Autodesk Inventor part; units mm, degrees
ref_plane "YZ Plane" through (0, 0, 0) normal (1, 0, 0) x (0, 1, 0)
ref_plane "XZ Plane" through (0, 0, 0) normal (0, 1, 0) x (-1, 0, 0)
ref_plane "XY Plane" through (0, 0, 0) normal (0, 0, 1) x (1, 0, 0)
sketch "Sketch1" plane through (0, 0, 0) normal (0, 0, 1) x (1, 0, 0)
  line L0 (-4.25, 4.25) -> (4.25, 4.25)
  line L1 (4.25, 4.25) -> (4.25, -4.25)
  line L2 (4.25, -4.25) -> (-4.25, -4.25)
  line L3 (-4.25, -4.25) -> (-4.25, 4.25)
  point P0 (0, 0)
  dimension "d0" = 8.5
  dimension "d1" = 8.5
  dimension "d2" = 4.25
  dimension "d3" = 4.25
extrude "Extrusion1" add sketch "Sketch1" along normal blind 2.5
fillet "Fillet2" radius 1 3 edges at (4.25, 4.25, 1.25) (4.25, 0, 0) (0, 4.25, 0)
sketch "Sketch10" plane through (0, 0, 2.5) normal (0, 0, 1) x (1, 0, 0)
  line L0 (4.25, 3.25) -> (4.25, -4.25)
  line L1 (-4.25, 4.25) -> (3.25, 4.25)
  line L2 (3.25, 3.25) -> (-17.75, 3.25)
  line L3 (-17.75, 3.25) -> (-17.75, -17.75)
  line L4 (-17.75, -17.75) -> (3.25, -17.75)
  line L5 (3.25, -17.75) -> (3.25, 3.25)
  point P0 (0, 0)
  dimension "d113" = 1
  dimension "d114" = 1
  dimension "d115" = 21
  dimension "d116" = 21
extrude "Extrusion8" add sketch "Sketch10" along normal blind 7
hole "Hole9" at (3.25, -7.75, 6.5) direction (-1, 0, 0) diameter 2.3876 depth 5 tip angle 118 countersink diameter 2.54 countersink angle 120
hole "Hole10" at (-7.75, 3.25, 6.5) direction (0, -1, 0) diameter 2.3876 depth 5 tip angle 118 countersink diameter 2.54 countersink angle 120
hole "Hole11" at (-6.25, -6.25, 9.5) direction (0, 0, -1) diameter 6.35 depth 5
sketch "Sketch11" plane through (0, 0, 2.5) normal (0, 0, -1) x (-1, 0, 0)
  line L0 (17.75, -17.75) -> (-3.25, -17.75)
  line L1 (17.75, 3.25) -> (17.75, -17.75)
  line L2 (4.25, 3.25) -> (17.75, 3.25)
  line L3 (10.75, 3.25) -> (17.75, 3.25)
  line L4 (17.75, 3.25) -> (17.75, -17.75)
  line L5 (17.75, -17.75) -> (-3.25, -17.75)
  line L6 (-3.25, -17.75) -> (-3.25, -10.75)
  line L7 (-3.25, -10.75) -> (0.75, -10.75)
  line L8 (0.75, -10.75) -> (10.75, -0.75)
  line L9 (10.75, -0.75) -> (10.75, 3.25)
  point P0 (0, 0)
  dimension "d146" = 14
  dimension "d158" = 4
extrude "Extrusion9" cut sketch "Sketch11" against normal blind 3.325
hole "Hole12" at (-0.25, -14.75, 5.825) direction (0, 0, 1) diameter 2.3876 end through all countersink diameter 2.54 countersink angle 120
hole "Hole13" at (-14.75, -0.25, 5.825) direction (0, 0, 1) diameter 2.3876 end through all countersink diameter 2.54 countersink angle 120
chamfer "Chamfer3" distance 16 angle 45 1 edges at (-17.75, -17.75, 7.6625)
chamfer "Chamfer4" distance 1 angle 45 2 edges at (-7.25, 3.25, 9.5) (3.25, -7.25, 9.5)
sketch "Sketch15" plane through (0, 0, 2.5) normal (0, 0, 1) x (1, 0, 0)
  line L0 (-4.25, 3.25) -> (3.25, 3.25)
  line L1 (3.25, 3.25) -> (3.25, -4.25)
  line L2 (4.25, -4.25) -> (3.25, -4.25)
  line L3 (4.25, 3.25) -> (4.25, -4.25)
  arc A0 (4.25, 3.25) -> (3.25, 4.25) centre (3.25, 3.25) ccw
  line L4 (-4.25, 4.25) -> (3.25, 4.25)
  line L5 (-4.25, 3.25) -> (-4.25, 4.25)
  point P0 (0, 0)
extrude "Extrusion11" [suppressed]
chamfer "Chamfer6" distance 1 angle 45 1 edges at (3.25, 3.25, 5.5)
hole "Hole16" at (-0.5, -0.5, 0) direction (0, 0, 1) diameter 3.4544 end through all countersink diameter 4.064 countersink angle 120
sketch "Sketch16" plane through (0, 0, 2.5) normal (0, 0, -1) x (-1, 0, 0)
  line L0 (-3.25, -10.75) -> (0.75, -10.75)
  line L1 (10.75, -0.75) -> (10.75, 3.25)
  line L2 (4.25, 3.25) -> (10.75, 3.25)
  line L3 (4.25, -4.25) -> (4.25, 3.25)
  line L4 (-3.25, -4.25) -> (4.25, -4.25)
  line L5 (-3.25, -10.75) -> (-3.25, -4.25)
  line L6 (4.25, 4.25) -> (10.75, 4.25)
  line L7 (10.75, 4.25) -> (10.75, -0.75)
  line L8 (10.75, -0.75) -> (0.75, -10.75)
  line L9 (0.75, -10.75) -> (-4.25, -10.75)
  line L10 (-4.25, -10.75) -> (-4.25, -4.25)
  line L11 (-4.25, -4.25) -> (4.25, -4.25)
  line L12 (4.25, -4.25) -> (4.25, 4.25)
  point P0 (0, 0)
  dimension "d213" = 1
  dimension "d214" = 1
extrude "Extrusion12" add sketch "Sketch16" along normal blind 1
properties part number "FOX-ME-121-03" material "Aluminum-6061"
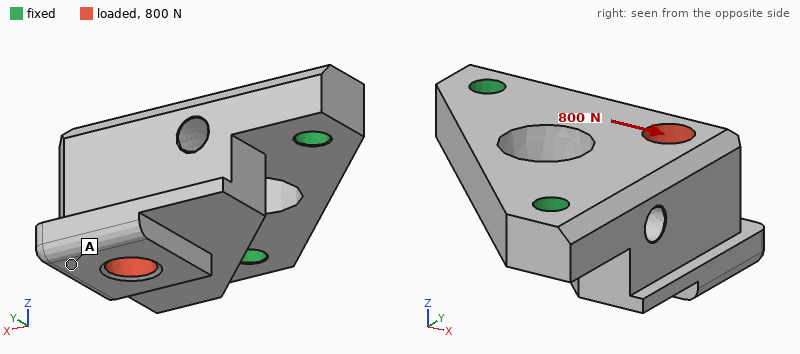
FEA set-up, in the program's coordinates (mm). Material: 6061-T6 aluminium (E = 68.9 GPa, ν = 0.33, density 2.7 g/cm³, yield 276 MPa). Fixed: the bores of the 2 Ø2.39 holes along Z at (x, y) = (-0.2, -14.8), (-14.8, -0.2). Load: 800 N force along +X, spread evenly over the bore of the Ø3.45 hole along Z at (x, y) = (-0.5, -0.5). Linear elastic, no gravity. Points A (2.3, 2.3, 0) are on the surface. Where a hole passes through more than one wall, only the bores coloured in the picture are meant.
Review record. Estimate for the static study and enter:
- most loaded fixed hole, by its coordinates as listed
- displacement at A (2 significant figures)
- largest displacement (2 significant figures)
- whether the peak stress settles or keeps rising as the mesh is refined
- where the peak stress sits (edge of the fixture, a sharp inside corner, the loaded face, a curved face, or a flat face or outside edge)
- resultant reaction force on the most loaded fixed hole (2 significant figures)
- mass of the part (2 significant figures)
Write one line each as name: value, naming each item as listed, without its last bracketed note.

most loaded fixed hole, by its coordinates as listed: (-14.8, -0.2)
displacement at A: 34 µm
largest displacement: 37 µm
whether the peak stress settles or keeps rising as the mesh is refined: keeps rising
where the peak stress sits: edge of the fixture
resultant reaction force on the most loaded fixed hole: 680 N
mass of the part: 4.3 g
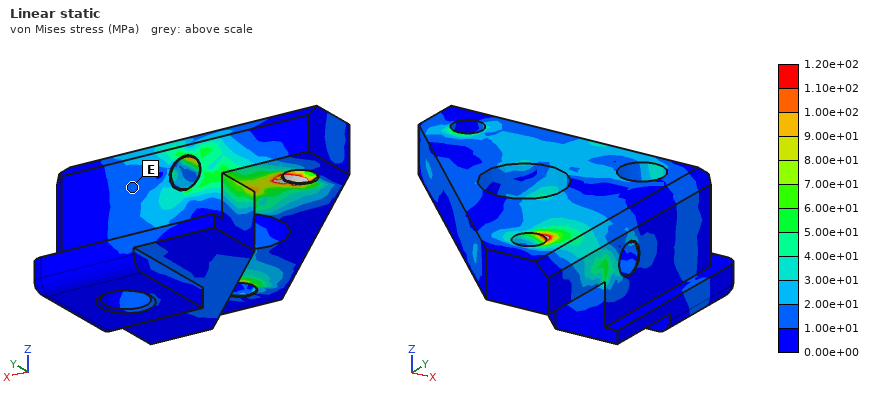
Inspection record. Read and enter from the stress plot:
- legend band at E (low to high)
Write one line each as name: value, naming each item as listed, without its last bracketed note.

legend band at E: 1.00e+01 to 2.00e+01 MPa
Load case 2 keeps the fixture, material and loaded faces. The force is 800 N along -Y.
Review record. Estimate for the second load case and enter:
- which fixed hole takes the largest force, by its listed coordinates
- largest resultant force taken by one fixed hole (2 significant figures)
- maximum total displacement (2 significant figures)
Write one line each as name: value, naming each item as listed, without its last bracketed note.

which fixed hole takes the largest force, by its listed coordinates: (-0.2, -14.8)
largest resultant force taken by one fixed hole: 680 N
maximum total displacement: 37 µm
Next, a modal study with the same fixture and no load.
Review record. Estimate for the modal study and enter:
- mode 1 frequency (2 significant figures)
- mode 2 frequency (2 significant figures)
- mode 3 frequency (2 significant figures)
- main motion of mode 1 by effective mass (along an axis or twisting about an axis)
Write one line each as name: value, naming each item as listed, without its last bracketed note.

mode 1 frequency: 10 kHz
mode 2 frequency: 36 kHz
mode 3 frequency: 37 kHz
main motion of mode 1 by effective mass: along Z
